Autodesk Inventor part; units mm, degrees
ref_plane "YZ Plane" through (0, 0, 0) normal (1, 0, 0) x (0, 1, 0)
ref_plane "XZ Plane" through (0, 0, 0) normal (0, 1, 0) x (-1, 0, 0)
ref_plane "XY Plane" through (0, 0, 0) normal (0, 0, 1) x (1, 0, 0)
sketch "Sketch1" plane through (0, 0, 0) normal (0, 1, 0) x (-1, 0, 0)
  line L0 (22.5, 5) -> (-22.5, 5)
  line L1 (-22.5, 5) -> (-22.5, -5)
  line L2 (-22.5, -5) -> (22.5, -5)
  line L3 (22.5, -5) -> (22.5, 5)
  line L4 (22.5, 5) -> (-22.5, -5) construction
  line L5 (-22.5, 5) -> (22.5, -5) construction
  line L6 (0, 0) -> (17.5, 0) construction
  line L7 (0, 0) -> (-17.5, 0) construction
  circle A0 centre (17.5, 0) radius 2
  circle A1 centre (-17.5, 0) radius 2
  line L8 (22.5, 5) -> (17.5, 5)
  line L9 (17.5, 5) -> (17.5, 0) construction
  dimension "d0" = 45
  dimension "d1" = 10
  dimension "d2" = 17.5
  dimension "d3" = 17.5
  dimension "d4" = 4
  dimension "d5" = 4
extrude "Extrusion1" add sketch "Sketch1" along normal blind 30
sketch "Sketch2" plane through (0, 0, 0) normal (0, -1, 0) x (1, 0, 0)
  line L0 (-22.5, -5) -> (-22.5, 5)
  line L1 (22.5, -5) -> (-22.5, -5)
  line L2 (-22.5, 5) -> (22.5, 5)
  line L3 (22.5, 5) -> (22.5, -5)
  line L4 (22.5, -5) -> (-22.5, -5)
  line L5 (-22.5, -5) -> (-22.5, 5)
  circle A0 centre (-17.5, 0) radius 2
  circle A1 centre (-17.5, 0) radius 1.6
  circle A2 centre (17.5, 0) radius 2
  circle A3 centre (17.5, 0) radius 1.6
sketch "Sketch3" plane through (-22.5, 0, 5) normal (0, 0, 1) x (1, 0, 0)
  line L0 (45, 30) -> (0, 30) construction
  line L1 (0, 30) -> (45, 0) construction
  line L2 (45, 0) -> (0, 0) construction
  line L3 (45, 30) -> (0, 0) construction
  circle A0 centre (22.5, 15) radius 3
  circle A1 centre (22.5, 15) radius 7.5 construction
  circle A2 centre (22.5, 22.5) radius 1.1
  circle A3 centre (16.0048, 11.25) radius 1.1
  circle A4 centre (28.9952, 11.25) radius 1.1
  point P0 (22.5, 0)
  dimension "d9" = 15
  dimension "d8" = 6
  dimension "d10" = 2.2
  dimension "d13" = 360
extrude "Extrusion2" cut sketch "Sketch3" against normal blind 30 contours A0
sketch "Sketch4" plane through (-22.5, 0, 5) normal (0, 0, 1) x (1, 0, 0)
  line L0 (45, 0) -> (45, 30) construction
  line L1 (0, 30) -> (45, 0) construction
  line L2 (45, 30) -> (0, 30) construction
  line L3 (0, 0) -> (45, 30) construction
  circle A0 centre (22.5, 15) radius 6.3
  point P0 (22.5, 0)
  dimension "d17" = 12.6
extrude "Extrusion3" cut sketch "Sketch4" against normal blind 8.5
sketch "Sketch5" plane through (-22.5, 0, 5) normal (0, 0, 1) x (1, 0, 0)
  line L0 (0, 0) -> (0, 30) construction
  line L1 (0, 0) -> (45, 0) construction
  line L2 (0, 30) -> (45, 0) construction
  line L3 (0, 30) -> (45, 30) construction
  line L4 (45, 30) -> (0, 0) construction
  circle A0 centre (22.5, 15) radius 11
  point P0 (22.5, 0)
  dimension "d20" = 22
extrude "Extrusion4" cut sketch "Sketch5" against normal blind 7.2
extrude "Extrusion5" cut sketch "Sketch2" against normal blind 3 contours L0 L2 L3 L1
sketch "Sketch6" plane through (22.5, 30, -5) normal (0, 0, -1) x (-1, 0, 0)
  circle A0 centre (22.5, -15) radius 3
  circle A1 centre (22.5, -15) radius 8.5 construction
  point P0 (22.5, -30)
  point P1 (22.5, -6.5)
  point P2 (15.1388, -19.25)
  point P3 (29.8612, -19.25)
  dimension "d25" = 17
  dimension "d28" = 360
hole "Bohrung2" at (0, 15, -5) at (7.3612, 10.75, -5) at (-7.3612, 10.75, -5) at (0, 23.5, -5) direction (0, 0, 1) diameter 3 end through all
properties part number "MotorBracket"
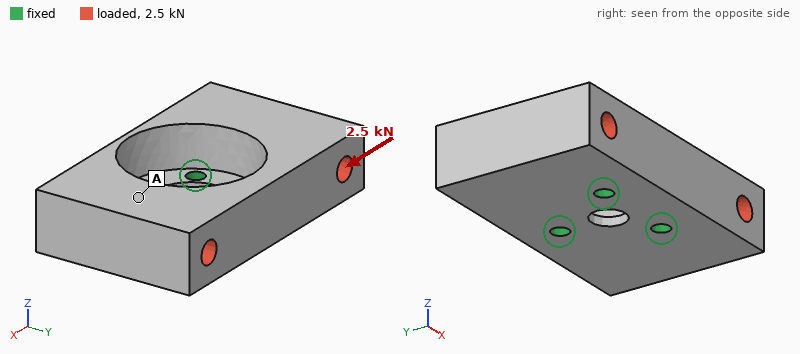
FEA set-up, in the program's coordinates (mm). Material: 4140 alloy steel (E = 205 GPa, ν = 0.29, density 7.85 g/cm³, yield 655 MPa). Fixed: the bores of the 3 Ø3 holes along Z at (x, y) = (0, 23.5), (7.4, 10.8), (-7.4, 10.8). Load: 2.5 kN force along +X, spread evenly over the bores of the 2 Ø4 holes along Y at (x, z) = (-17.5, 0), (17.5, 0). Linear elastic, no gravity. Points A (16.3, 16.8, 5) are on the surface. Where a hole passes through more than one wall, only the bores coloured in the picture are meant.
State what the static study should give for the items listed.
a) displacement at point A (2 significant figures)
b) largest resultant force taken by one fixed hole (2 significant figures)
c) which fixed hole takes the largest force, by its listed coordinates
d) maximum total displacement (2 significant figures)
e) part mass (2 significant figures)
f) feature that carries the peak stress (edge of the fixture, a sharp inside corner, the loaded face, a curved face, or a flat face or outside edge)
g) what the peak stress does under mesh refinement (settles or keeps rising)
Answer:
7.3 µm
1.2 kN
(0, 23.5)
11 µm
66 g
edge of the fixture
keeps rising
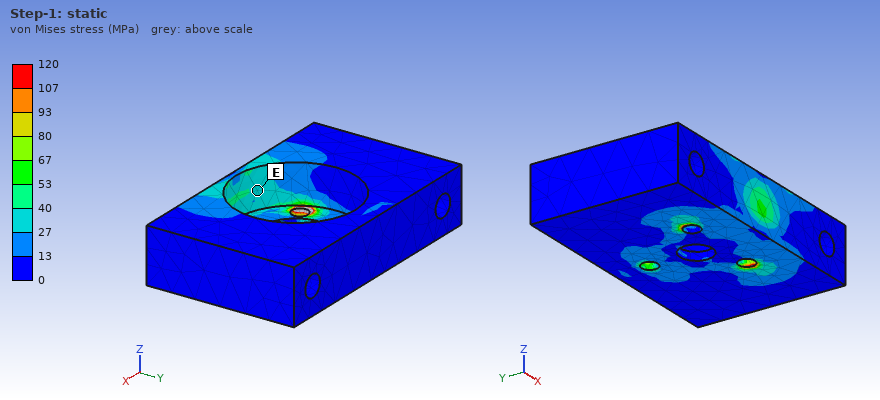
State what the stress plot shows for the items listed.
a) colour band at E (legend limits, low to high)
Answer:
27 to 40 MPa
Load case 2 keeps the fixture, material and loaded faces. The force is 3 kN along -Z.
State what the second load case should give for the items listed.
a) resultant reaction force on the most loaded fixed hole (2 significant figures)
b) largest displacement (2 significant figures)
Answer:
1.2 kN
21 µm
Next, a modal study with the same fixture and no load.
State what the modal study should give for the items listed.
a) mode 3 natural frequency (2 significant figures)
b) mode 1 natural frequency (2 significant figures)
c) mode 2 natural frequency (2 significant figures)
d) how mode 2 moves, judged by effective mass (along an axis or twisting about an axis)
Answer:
15 kHz
7300 Hz
11 kHz
along Z
